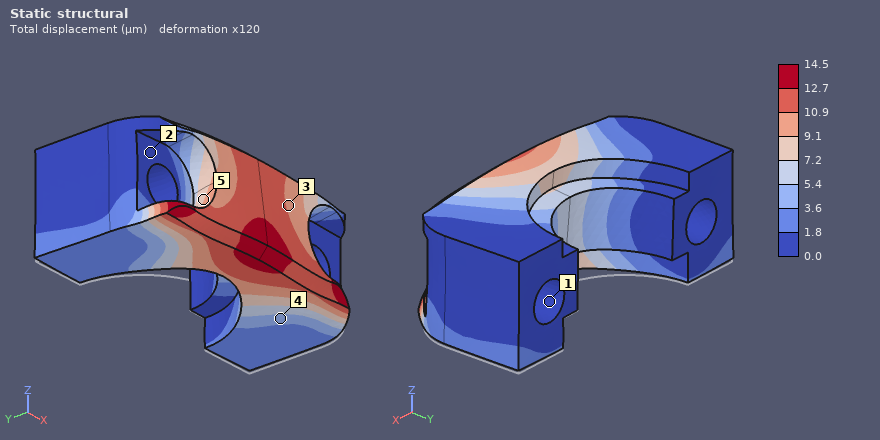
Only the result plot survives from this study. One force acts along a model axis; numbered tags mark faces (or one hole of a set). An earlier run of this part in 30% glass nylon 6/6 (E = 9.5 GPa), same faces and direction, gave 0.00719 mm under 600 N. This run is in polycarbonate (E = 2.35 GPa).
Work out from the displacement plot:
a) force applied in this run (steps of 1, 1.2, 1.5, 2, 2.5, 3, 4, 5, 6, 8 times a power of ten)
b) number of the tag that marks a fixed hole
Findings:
300 N
1
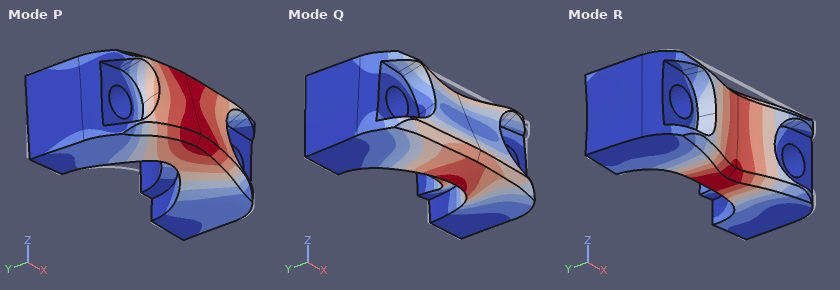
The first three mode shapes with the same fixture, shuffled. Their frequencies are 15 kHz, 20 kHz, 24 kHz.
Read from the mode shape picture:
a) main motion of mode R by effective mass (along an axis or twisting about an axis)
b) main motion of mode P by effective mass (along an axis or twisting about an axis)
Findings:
along Y
along Z
